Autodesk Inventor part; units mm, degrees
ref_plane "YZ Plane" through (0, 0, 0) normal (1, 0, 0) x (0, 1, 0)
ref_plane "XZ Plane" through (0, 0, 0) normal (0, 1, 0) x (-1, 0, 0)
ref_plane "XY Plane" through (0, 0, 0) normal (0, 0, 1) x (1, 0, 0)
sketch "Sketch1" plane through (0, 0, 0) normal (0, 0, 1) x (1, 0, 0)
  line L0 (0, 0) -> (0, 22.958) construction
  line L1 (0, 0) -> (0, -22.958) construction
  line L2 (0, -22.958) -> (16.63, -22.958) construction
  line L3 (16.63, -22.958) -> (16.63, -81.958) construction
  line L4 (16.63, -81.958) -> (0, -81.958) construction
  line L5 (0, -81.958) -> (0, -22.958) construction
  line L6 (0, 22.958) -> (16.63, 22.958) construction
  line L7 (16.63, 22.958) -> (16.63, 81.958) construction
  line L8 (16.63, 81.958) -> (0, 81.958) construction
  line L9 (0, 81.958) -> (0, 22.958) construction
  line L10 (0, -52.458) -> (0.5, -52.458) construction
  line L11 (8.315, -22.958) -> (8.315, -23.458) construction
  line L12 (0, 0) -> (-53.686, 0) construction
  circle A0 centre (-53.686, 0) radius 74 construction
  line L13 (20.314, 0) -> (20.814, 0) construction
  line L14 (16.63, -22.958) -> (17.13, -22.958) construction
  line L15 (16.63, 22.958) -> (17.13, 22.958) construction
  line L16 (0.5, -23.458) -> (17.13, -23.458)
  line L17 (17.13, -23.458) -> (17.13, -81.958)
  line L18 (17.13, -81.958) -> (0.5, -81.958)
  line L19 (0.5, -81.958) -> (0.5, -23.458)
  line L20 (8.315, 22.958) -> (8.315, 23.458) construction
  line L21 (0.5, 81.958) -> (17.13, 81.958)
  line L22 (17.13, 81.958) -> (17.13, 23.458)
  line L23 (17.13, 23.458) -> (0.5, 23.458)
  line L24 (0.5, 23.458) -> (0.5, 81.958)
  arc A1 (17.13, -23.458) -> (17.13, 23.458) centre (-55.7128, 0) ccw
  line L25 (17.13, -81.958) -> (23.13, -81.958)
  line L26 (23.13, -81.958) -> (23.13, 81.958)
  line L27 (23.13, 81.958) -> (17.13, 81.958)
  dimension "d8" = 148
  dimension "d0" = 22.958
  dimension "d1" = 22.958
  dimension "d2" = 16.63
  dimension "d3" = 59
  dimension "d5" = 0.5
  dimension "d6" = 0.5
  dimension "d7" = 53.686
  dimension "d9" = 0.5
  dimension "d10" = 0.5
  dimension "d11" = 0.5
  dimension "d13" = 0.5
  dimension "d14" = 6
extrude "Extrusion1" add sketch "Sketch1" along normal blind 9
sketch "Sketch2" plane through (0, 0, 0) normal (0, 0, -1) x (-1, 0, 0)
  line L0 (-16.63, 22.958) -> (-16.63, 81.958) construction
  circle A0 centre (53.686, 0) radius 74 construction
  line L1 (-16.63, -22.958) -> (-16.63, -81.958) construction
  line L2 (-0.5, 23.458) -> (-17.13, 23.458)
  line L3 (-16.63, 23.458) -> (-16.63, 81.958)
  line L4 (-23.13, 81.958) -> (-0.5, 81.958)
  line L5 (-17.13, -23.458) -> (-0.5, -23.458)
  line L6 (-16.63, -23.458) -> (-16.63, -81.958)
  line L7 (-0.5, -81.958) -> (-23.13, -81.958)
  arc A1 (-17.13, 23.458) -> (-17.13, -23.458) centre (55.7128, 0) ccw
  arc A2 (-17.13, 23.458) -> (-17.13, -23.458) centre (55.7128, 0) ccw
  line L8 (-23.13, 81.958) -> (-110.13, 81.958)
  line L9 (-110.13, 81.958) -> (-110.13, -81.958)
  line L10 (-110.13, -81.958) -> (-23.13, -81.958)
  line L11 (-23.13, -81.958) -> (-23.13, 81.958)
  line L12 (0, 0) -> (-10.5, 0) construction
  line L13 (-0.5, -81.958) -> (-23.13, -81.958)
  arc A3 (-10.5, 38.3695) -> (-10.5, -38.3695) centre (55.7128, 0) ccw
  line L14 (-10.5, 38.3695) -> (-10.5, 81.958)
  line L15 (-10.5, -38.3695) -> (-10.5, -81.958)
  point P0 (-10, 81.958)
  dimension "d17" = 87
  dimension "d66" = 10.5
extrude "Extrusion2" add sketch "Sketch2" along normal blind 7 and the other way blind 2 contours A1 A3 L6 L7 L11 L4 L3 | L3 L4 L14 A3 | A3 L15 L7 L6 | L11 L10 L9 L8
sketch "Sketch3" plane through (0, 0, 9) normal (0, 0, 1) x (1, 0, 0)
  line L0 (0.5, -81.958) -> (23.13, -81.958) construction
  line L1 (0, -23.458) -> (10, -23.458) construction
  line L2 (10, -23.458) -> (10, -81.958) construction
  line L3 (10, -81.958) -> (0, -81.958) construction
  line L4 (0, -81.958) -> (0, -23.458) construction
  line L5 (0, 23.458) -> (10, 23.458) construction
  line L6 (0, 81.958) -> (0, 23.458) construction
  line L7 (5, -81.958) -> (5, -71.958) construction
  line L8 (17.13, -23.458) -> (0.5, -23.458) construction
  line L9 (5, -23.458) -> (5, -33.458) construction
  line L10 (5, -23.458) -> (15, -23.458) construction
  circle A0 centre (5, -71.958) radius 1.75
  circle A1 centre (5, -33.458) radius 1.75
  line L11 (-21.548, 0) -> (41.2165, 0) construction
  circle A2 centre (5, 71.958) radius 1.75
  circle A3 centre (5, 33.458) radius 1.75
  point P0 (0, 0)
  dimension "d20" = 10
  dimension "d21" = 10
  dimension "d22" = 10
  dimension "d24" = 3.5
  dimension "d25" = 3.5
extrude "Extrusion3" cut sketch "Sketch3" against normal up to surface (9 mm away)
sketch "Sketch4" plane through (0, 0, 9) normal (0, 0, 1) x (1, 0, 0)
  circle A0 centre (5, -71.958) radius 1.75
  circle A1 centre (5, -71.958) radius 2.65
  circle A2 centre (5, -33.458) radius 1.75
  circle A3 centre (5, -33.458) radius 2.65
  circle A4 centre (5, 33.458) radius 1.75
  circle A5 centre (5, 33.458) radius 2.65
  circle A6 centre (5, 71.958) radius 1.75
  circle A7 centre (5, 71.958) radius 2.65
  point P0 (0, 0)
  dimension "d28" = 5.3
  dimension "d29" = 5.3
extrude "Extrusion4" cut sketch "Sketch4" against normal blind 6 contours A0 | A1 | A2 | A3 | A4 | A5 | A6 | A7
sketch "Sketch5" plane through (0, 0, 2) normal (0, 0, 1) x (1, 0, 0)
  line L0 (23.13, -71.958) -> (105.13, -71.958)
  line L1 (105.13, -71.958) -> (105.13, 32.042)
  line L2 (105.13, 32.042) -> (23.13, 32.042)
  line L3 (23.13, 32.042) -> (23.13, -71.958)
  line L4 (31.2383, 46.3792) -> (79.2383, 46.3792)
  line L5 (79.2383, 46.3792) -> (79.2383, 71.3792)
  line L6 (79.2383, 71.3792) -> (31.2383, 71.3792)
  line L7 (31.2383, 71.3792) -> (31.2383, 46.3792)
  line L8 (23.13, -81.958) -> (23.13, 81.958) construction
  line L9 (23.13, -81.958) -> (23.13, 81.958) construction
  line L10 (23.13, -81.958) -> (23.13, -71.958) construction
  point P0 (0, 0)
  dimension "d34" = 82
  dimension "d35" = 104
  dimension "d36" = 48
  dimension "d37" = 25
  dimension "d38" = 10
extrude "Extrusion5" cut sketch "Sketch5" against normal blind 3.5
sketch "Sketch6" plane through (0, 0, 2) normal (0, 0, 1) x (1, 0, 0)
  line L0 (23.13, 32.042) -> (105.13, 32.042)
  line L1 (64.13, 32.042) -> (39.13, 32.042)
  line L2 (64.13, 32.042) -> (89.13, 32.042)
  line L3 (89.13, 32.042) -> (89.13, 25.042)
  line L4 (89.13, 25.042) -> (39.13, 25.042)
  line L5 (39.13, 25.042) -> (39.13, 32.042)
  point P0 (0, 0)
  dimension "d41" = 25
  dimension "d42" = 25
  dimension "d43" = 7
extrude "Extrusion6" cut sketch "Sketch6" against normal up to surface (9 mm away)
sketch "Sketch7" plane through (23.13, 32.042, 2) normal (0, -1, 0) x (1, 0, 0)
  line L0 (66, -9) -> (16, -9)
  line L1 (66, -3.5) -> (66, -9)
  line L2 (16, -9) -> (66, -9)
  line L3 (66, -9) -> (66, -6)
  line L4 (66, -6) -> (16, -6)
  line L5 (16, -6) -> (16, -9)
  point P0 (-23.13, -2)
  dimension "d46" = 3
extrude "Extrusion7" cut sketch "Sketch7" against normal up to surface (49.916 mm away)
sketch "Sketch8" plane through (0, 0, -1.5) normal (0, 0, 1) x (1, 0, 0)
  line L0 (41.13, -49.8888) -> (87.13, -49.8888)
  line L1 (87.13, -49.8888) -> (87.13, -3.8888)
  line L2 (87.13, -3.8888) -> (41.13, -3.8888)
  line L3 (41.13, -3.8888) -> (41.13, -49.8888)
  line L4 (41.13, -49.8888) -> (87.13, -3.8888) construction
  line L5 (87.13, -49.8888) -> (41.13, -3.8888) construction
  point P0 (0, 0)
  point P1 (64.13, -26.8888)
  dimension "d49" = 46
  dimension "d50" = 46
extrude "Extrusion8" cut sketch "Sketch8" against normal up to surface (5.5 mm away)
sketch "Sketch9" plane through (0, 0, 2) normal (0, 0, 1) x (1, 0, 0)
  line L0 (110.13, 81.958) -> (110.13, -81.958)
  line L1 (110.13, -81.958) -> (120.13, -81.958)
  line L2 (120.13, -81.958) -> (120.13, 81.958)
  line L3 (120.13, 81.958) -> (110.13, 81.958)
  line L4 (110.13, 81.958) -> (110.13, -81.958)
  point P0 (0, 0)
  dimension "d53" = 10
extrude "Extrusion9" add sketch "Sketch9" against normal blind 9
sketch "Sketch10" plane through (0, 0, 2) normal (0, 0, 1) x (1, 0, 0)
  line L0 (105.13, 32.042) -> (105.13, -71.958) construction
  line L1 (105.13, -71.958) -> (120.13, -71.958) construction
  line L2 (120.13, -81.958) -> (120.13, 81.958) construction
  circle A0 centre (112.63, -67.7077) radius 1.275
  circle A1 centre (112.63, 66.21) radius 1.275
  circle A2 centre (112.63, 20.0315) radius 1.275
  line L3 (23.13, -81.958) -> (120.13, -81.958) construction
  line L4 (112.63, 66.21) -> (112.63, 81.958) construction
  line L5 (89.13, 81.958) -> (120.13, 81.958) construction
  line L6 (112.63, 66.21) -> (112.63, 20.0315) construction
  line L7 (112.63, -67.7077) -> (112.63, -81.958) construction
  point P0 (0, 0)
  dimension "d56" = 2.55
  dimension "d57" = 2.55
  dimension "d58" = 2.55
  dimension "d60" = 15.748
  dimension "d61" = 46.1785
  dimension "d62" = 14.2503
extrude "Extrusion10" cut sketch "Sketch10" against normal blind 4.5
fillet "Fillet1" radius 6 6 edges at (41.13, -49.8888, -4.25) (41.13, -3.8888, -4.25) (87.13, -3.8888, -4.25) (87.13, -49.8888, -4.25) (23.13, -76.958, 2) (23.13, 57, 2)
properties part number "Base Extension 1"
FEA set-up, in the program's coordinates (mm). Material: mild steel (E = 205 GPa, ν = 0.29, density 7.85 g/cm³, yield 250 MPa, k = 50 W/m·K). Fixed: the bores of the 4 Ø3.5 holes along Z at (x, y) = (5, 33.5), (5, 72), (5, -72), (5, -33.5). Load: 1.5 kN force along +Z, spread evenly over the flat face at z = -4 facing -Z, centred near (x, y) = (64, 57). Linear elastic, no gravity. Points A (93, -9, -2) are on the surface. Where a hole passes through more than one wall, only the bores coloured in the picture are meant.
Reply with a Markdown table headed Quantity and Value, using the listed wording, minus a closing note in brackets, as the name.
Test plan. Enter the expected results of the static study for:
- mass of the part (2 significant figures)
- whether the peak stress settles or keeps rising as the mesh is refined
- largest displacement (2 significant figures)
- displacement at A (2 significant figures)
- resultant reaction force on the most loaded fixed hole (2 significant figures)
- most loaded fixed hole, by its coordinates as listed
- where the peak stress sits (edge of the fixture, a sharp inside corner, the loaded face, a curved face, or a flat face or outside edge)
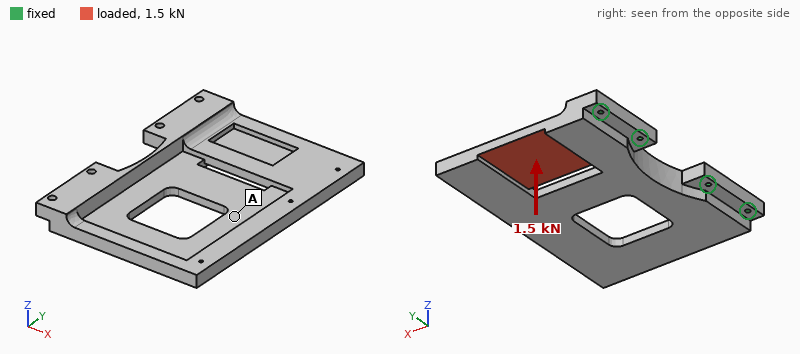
| Quantity | Value |
|---|---|
| mass of the part | 970 g |
| whether the peak stress settles or keeps rising as the mesh is refined | keeps rising |
| largest displacement | 0.91 mm |
| displacement at A | 0.47 mm |
| resultant reaction force on the most loaded fixed hole | 1.3 kN |
| most loaded fixed hole, by its coordinates as listed | (5, 72) |
| where the peak stress sits | edge of the fixture |
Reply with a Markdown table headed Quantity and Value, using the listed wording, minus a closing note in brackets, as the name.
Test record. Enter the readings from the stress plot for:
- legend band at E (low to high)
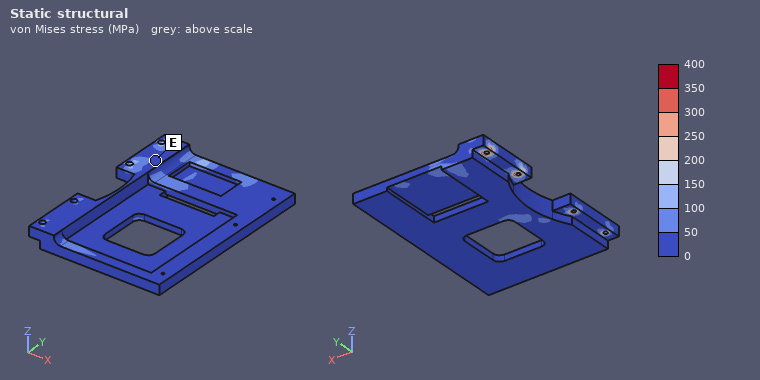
| Quantity | Value |
|---|---|
| legend band at E | 0 to 50 MPa |
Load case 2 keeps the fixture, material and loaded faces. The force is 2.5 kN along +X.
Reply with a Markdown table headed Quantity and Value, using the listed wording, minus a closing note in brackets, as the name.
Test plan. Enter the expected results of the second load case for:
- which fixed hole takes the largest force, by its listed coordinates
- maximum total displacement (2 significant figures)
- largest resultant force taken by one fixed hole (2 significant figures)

| Quantity | Value |
|---|---|
| which fixed hole takes the largest force, by its listed coordinates | (5, 72) |
| maximum total displacement | 0.15 mm |
| largest resultant force taken by one fixed hole | 1.6 kN |
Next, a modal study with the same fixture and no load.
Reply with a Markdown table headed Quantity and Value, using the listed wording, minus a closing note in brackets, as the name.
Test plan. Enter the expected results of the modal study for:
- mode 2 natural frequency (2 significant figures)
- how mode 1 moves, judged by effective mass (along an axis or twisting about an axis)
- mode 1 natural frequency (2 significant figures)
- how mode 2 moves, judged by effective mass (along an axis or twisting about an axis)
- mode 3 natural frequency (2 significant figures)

| Quantity | Value |
|---|---|
| mode 2 natural frequency | 650 Hz |
| how mode 1 moves, judged by effective mass | along Z |
| mode 1 natural frequency | 280 Hz |
| how mode 2 moves, judged by effective mass | twisting about X |
| mode 3 natural frequency | 1700 Hz |
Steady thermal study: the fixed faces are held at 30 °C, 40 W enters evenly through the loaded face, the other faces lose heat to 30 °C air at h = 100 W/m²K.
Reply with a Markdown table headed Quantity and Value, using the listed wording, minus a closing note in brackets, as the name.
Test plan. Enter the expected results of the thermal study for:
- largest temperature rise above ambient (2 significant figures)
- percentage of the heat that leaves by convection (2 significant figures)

| Quantity | Value |
|---|---|
| largest temperature rise above ambient | 42 K |
| percentage of the heat that leaves by convection | 81 % |
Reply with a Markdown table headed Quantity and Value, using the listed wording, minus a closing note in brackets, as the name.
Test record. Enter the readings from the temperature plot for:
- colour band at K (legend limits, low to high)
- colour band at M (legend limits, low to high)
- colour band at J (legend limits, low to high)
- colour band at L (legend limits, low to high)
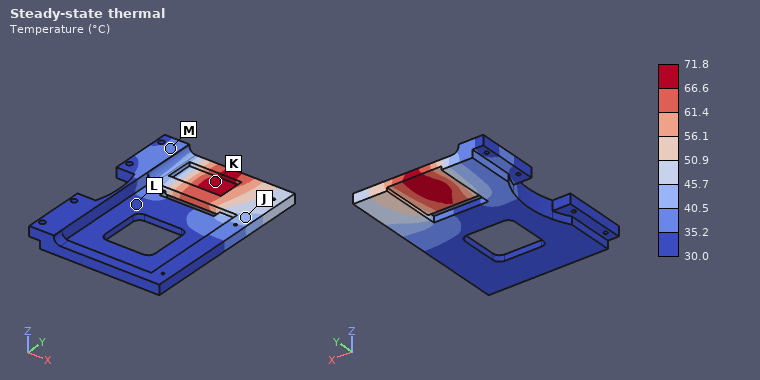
| Quantity | Value |
|---|---|
| colour band at K | 66.6 to 71.8 °C |
| colour band at M | 35.2 to 40.5 °C |
| colour band at J | 40.5 to 45.7 °C |
| colour band at L | 30.0 to 35.2 °C |
